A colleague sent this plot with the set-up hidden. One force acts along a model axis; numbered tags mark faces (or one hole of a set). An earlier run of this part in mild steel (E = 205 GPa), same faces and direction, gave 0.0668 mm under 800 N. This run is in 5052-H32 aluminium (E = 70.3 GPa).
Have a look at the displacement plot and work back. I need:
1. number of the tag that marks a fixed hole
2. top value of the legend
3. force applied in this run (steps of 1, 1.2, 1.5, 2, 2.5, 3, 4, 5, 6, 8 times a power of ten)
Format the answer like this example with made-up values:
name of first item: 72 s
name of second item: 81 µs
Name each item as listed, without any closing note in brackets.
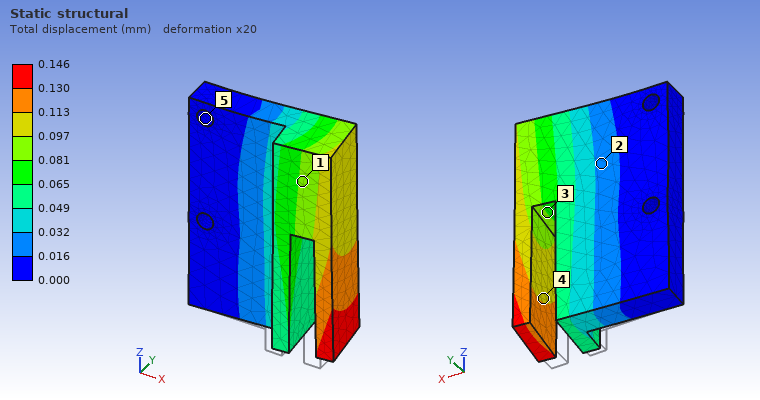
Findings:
number of the tag that marks a fixed hole: 5
top value of the legend: 0.146 mm
force applied in this run: 600 N
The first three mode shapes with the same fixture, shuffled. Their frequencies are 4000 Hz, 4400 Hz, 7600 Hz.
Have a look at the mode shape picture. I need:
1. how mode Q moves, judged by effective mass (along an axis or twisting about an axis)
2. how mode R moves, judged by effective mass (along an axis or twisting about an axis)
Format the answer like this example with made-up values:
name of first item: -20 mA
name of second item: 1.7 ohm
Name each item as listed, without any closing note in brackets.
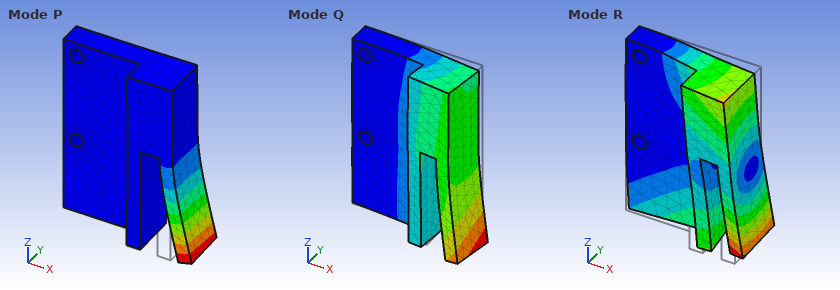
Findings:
how mode Q moves, judged by effective mass: along Y
how mode R moves, judged by effective mass: twisting about X
